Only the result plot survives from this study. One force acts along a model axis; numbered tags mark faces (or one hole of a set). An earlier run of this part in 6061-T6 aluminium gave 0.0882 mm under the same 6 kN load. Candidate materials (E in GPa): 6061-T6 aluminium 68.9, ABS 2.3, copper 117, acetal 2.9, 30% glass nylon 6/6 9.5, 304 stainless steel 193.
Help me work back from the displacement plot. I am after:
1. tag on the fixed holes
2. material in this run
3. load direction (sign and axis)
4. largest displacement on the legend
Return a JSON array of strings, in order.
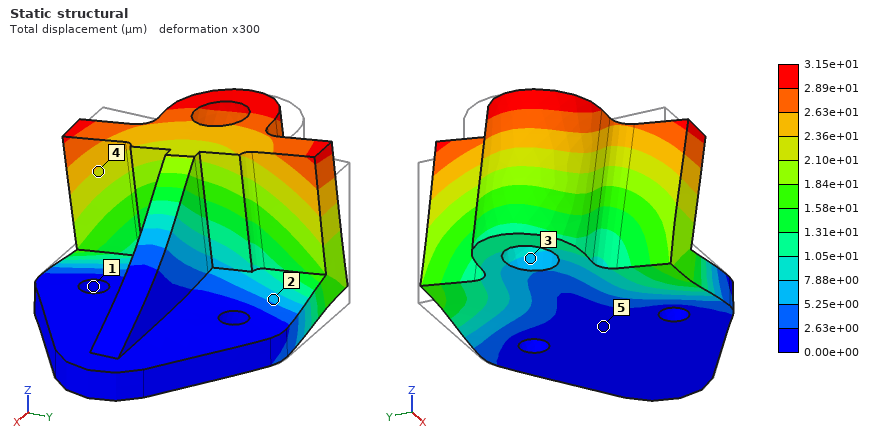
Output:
["1", "304 stainless steel", "-Y", "3.15e+01 µm"]
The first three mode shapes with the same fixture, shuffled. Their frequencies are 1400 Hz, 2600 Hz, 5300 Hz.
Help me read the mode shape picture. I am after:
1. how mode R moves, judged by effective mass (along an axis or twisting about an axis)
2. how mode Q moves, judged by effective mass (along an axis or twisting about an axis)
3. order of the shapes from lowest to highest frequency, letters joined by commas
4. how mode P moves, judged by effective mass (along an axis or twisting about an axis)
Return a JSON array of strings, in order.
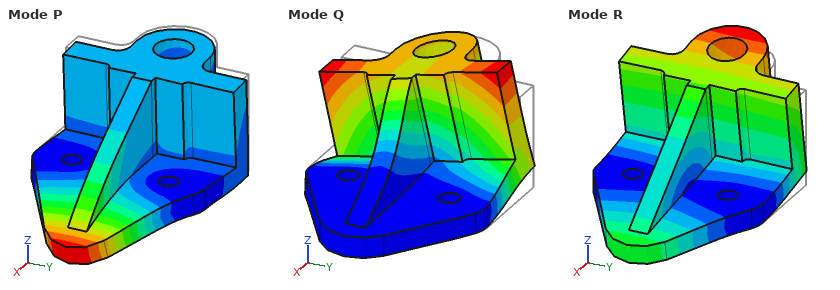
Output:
["along Z", "along Y", "R, Q, P", "along Z"]
